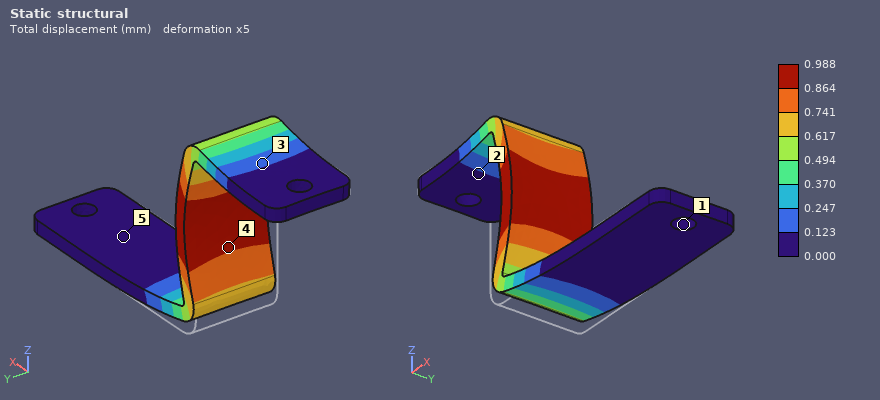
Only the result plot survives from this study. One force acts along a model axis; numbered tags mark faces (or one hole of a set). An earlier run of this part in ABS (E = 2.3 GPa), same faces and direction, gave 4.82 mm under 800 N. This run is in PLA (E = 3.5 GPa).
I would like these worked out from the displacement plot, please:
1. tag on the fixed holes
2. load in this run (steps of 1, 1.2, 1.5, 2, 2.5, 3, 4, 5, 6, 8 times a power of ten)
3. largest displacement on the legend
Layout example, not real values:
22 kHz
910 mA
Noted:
1
250 N
0.988 mm
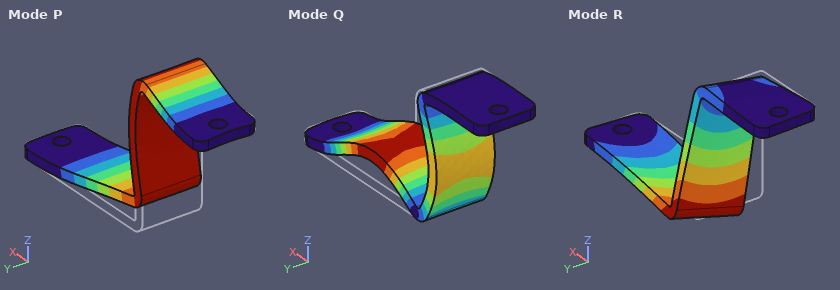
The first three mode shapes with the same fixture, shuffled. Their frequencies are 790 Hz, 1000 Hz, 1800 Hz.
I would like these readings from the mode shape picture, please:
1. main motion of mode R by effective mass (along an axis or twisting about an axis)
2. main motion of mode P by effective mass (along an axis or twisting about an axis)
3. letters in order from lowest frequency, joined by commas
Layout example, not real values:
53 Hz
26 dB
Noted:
along Y
along Z
P, R, Q
